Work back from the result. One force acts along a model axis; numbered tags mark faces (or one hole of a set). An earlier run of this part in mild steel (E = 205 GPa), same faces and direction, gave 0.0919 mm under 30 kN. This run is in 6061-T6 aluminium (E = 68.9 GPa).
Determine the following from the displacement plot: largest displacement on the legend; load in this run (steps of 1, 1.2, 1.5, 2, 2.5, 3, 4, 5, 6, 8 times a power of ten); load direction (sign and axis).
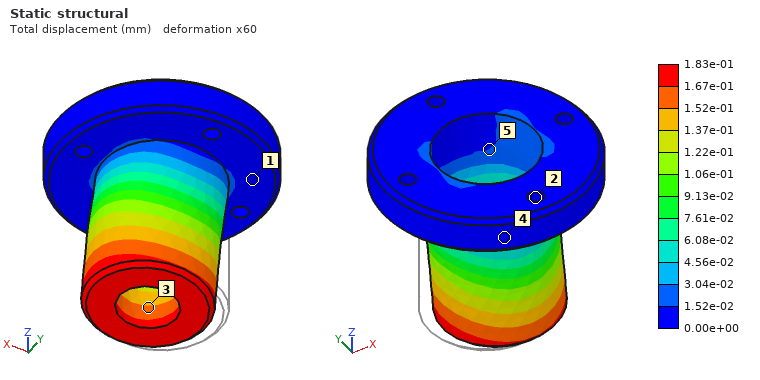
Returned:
1.83e-01 mm
20 kN
+X
